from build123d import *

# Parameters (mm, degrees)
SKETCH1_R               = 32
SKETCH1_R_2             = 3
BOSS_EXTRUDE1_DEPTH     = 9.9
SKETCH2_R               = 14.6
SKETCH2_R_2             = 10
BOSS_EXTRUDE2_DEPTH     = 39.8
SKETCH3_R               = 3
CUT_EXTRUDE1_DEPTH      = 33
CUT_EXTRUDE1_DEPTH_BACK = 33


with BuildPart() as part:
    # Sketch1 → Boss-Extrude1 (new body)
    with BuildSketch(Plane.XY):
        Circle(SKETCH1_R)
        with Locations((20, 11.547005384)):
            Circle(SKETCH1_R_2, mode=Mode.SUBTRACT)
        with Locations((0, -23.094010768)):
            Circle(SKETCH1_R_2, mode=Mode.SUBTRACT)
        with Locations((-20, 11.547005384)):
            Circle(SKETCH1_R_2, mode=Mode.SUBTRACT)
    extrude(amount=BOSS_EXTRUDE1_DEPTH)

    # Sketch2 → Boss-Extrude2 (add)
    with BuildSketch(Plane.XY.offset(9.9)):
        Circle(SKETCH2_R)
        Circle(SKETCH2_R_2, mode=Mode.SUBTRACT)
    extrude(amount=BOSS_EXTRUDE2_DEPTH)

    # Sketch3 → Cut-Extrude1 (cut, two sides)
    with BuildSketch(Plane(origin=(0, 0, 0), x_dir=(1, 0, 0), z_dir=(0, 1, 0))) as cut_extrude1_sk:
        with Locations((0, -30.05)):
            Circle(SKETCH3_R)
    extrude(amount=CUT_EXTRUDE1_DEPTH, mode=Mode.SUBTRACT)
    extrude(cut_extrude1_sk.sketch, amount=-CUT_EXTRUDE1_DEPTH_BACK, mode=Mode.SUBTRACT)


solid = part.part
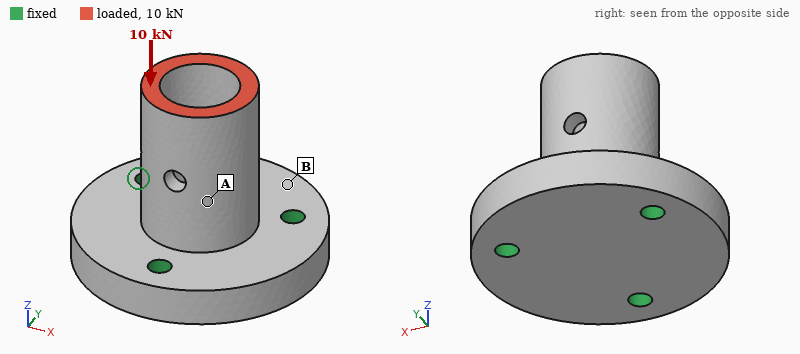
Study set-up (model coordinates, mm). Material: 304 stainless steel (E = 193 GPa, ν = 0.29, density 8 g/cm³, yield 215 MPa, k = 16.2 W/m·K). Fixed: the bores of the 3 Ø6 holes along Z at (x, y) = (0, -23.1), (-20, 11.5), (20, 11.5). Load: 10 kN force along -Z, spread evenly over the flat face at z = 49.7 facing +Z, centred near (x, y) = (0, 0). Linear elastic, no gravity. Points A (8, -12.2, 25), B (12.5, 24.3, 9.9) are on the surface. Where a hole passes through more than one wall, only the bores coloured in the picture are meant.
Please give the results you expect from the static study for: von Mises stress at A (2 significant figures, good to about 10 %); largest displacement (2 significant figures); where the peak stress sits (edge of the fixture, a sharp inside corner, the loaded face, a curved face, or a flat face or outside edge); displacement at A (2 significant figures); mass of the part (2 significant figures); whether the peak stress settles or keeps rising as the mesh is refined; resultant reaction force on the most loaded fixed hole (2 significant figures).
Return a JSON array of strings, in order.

["33 MPa", "11 µm", "edge of the fixture", "6.4 µm", "360 g", "keeps rising", "3.4 kN"]
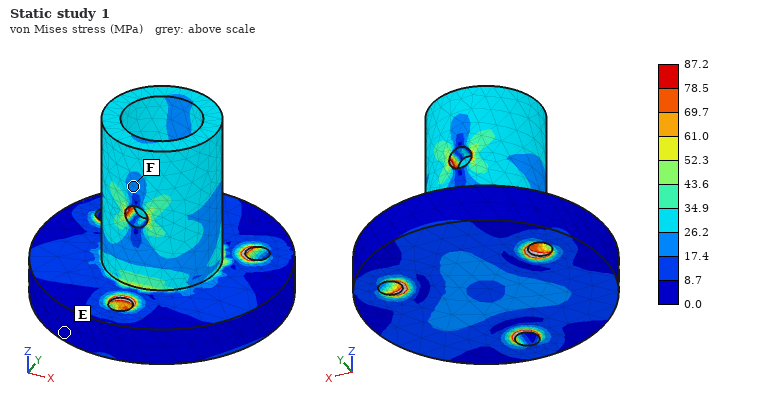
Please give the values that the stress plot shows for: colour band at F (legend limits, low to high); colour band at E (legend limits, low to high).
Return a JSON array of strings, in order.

["17.4 to 26.2 MPa", "0.0 to 8.7 MPa"]
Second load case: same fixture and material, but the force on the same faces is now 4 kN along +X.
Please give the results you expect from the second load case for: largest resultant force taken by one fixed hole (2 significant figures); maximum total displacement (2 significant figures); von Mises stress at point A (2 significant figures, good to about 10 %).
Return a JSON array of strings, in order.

["4.6 kN", "51 µm", "39 MPa"]
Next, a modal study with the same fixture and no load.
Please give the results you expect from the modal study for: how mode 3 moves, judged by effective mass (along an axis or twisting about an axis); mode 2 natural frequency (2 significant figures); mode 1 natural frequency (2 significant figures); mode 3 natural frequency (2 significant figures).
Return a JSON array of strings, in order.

["along Z", "7500 Hz", "7400 Hz", "15 kHz"]
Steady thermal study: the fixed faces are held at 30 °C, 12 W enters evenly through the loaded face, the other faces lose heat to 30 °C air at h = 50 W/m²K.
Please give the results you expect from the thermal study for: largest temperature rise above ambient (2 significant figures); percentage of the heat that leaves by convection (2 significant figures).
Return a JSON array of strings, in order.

["54 K", "70 %"]
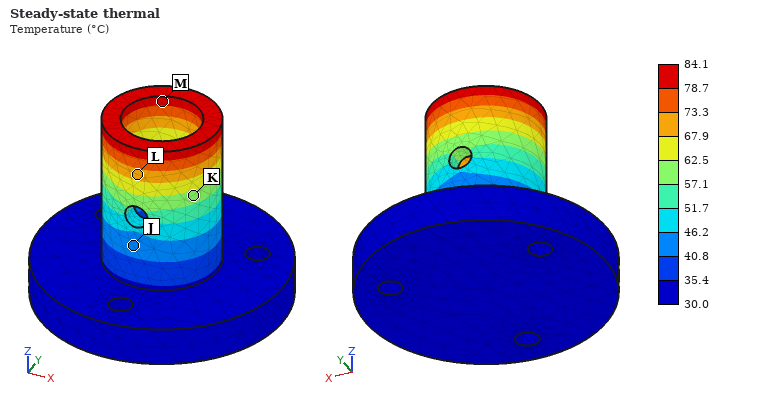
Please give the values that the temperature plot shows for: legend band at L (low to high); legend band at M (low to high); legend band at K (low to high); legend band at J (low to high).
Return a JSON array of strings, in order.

["67.9 to 73.3 °C", "78.7 to 84.1 °C", "57.1 to 62.5 °C", "40.8 to 46.2 °C"]
